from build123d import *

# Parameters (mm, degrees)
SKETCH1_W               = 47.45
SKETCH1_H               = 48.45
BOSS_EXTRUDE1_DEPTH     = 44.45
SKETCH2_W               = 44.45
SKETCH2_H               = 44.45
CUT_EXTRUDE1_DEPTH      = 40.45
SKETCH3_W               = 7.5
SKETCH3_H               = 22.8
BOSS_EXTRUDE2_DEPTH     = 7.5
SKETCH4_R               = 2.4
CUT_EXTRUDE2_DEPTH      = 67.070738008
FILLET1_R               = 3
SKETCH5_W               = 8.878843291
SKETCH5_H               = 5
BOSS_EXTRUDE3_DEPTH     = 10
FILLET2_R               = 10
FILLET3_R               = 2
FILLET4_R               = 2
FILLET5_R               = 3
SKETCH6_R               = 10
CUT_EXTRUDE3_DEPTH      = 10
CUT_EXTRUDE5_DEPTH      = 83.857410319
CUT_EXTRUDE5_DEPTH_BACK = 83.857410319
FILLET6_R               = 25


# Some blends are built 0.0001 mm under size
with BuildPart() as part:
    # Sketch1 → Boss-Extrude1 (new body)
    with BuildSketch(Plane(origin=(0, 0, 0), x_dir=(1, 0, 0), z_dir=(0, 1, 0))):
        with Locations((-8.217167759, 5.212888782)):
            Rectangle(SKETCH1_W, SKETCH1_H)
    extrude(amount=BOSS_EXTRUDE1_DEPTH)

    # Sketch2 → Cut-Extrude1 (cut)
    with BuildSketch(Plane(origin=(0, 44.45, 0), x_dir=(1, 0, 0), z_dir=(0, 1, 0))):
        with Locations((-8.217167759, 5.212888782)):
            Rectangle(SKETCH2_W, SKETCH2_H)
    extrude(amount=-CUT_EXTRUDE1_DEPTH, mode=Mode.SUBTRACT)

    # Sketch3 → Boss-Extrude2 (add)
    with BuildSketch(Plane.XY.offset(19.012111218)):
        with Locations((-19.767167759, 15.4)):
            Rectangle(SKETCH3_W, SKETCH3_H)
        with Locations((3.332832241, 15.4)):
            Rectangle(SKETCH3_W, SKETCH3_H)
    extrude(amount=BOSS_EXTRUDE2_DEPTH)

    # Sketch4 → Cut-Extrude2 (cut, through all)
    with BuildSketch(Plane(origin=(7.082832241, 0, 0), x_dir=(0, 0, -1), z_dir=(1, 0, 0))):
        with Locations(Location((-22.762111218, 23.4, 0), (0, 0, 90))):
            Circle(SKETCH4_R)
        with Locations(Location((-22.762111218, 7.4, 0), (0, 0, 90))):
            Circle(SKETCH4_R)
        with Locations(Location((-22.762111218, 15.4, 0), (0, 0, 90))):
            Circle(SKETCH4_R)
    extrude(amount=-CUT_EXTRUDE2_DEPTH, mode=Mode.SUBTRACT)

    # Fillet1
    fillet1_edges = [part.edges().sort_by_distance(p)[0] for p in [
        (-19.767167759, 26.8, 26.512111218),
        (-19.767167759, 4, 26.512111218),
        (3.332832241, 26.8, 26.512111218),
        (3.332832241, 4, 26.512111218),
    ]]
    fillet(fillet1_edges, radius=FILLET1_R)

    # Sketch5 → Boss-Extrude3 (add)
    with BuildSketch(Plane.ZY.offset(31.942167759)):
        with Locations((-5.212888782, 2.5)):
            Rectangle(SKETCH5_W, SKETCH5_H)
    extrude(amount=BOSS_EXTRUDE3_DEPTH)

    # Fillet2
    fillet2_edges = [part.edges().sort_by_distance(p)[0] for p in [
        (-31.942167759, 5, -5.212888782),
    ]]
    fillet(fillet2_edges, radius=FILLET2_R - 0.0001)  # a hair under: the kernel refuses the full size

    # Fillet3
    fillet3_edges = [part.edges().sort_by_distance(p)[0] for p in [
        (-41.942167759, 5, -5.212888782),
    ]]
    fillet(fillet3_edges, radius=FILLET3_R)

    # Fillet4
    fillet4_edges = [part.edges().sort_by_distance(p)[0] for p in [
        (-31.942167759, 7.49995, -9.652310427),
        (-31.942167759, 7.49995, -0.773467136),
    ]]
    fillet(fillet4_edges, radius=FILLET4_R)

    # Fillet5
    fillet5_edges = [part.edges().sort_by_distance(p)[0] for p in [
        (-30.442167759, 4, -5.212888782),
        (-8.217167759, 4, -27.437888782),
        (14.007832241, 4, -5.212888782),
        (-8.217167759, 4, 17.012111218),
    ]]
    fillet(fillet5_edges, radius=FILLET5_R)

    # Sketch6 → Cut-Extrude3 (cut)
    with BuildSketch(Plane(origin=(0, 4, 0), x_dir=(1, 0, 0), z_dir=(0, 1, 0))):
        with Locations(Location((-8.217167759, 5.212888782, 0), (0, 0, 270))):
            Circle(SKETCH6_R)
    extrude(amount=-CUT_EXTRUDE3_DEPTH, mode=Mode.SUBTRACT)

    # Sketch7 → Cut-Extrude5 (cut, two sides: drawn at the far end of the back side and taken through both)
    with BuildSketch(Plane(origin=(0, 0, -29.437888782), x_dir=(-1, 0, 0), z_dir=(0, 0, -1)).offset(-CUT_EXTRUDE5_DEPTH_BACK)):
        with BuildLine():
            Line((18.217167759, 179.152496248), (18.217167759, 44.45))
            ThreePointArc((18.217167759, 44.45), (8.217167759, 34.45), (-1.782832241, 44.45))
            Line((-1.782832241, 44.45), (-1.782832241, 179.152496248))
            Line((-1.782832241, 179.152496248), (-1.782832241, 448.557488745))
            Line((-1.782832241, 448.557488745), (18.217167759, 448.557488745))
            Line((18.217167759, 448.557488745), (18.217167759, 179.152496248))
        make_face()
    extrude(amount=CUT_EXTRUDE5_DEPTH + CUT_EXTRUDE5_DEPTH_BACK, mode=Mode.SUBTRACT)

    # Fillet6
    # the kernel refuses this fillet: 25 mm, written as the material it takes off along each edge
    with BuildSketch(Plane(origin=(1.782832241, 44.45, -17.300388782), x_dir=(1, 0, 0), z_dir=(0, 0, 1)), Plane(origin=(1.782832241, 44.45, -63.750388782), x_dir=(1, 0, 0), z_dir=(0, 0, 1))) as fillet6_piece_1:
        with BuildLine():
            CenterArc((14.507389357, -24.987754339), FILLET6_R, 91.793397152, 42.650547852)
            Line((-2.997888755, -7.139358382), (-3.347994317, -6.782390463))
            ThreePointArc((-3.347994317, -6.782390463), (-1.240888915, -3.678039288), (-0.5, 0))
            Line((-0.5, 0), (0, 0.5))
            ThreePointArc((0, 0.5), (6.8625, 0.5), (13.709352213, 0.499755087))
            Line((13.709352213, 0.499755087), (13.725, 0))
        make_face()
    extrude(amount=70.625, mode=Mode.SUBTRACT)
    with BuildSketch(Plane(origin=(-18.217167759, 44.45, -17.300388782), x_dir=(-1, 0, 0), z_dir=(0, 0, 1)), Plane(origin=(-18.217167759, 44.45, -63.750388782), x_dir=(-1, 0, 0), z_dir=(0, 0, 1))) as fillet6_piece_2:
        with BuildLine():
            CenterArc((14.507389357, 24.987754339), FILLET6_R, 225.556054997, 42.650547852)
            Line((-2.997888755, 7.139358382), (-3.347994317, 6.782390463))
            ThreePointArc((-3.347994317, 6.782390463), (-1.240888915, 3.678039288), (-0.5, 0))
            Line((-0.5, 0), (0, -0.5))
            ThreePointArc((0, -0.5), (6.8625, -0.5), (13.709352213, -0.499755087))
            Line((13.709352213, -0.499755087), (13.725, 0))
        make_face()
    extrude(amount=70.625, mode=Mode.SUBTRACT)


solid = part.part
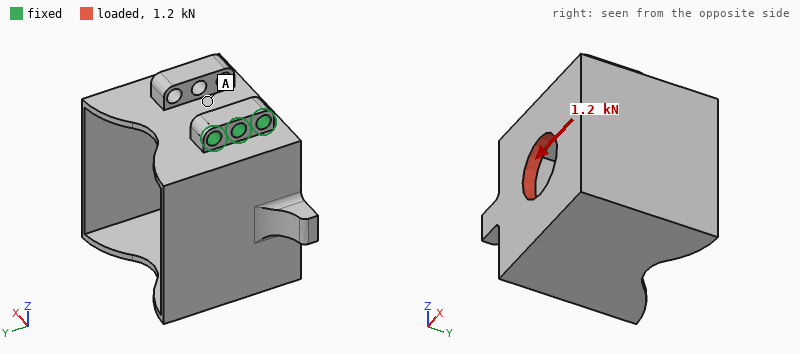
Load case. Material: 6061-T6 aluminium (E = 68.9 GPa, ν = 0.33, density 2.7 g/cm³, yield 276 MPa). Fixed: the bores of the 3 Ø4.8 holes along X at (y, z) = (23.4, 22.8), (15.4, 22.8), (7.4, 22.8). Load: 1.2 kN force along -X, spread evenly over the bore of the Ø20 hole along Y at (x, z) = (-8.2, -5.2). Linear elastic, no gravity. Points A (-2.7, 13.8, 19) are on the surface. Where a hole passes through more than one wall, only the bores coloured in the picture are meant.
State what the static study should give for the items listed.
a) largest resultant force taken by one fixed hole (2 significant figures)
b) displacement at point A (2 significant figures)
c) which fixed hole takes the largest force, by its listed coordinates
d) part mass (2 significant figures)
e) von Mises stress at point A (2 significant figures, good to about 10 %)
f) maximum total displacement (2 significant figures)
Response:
870 N
0.19 mm
(7.4, 22.8)
62 g
28 MPa
0.95 mm
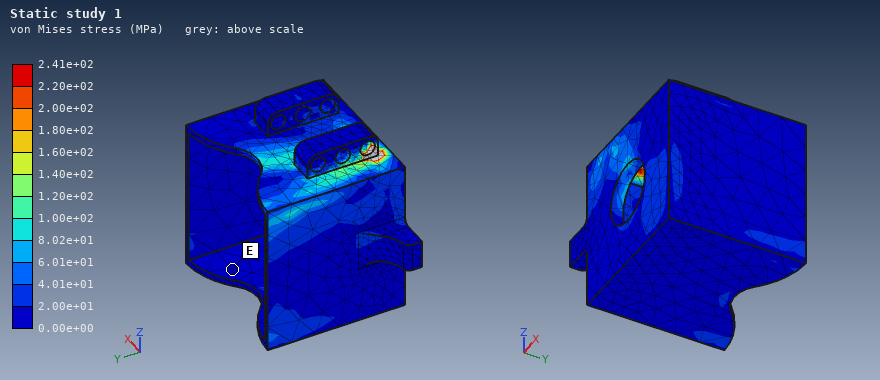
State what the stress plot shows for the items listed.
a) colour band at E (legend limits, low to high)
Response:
0.00e+00 to 2.00e+01 MPa
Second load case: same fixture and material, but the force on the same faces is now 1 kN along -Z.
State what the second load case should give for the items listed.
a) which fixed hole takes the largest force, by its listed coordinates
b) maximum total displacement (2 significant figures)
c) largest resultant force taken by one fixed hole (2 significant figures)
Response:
(7.4, 22.8)
0.39 mm
1.3 kN
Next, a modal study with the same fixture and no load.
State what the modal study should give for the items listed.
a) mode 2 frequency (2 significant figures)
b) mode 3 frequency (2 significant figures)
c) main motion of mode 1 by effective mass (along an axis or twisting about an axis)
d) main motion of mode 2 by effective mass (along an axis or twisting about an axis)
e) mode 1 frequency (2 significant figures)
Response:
870 Hz
1900 Hz
along X
along Y
770 Hz
